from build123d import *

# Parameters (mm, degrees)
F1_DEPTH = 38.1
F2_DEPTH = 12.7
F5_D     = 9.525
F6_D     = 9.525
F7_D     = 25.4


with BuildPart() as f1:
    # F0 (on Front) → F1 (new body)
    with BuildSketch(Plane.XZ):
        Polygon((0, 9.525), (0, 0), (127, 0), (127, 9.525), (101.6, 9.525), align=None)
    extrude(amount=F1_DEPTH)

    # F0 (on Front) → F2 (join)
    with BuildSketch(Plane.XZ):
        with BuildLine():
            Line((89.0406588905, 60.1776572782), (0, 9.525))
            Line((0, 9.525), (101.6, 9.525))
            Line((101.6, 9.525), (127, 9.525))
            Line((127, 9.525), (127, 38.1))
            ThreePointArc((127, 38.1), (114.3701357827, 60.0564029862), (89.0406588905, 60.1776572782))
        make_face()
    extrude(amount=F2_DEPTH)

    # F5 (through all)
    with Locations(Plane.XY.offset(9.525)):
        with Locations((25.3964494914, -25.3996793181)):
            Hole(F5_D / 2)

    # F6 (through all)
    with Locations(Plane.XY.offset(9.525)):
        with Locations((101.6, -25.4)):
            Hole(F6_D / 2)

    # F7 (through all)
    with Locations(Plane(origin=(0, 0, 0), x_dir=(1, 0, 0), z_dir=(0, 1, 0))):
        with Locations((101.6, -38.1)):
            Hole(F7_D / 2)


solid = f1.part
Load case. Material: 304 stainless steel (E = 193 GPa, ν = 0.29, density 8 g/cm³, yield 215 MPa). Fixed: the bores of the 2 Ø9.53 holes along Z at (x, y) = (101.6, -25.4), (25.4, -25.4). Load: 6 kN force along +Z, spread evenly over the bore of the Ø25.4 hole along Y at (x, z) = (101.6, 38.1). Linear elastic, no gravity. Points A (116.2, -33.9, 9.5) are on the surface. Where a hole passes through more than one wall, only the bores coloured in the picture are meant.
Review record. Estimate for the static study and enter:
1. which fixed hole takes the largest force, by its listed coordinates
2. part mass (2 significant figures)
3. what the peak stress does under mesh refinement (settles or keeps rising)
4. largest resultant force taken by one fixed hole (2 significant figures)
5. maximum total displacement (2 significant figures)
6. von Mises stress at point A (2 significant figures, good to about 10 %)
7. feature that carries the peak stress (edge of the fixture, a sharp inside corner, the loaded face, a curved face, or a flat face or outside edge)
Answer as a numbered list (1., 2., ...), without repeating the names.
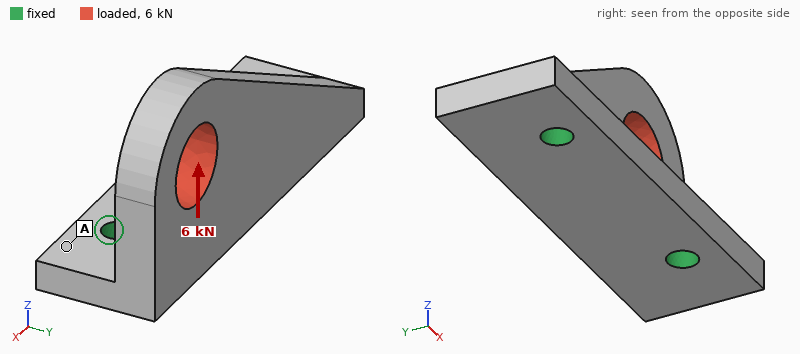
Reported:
1. (101.6, -25.4)
2. 730 g
3. keeps rising
4. 5.8 kN
5. 70 µm
6. 26 MPa
7. edge of the fixture
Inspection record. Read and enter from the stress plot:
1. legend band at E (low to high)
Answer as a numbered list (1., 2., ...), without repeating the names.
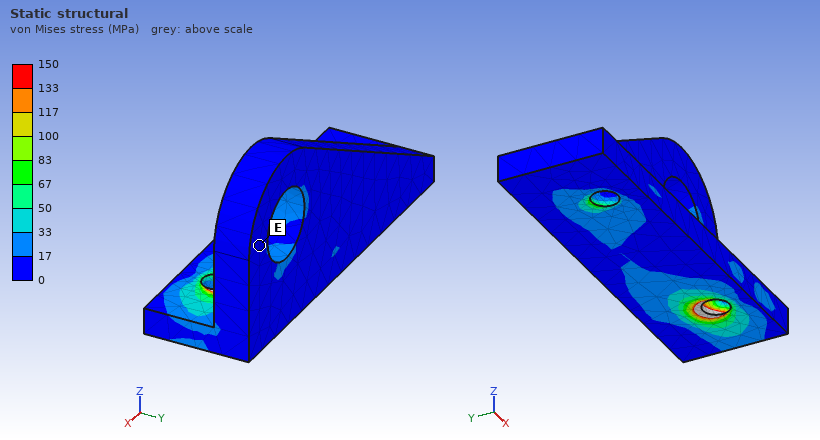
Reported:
1. 0 to 17 MPa
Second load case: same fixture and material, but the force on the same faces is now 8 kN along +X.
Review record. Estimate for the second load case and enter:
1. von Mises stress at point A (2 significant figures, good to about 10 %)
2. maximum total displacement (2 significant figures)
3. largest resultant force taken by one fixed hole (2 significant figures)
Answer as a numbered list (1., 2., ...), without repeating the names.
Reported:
1. 15 MPa
2. 33 µm
3. 5.5 kN
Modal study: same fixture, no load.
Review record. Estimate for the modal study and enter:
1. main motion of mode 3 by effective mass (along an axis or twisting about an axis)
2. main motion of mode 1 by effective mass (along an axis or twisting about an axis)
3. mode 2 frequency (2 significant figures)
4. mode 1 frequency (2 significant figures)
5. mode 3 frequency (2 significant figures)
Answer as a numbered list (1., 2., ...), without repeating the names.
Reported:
1. along Z
2. along Y
3. 4800 Hz
4. 2000 Hz
5. 6000 Hz
